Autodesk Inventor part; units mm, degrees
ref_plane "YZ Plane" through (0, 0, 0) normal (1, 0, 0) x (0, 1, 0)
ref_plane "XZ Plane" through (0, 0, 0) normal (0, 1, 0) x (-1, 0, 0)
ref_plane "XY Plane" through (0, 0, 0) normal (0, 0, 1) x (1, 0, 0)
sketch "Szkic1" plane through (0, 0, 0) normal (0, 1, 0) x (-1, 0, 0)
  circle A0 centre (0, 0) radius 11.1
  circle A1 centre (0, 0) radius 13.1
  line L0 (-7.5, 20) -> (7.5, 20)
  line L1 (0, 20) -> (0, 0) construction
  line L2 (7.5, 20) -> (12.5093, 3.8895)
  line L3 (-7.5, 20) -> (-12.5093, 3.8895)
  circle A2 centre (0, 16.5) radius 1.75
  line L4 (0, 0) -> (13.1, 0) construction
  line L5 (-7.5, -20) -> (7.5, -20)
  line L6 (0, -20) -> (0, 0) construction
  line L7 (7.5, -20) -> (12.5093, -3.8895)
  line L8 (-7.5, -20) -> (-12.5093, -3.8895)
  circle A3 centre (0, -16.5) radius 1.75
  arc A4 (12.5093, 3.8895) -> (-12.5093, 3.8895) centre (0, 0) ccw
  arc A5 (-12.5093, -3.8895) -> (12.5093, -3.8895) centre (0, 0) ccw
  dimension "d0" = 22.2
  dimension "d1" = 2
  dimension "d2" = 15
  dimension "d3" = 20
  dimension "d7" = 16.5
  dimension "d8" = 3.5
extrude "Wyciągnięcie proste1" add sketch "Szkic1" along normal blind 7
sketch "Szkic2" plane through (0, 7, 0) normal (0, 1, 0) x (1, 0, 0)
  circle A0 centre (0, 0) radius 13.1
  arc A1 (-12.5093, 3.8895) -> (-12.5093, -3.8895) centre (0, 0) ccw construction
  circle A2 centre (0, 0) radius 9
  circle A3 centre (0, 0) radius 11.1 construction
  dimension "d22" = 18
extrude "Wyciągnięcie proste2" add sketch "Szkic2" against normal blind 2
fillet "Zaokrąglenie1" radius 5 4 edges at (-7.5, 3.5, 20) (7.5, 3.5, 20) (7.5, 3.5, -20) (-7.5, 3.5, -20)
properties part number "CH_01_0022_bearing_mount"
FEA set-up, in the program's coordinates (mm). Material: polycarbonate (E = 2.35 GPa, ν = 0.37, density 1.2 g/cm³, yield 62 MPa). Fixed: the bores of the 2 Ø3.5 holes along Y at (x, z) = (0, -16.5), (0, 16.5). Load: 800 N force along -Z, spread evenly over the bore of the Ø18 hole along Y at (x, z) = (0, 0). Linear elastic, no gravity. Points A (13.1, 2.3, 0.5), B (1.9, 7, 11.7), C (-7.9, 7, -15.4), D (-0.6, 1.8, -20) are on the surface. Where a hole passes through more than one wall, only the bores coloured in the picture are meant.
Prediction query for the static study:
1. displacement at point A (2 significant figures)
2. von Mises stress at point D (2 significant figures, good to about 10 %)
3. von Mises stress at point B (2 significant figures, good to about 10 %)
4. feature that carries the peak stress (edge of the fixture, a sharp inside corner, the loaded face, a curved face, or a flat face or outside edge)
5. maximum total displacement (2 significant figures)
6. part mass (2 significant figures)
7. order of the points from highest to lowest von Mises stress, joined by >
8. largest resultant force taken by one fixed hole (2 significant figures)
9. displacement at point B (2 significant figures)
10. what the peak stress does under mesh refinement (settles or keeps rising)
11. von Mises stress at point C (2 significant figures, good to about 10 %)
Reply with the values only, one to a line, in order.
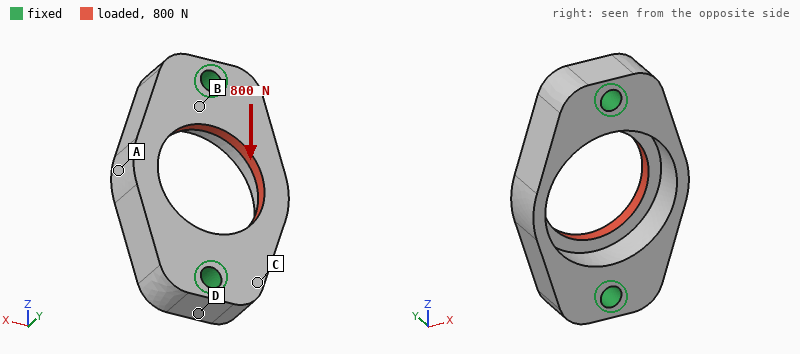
42 µm
8.9 MPa
13 MPa
edge of the fixture
95 µm
3.9 g
B > D > C > A
400 N
22 µm
keeps rising
4.1 MPa
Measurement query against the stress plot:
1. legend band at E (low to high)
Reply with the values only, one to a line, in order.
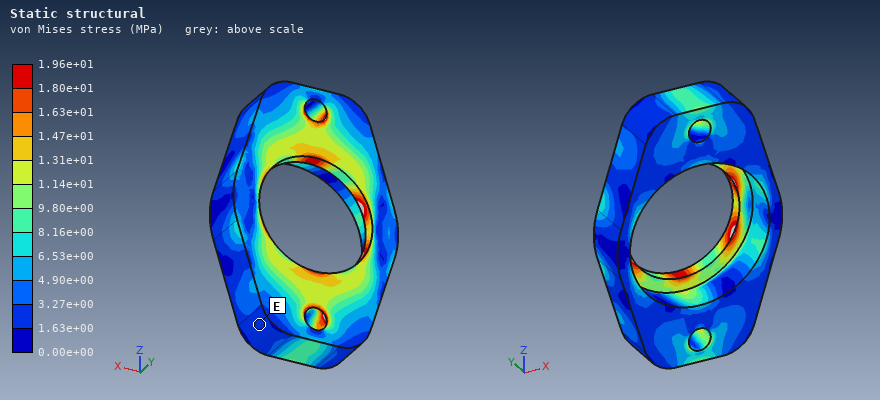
1.63e+00 to 3.27e+00 MPa
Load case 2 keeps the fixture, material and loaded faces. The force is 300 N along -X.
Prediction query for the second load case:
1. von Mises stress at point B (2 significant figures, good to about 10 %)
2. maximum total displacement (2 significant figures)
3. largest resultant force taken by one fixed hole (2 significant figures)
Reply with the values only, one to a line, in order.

5.4 MPa
87 µm
150 N
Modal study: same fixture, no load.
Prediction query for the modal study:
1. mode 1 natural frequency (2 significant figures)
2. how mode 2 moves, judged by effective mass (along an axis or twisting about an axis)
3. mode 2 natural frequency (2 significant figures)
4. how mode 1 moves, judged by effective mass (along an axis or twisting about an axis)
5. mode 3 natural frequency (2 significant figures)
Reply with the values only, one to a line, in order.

5900 Hz
along Y
6400 Hz
twisting about Z
7800 Hz
